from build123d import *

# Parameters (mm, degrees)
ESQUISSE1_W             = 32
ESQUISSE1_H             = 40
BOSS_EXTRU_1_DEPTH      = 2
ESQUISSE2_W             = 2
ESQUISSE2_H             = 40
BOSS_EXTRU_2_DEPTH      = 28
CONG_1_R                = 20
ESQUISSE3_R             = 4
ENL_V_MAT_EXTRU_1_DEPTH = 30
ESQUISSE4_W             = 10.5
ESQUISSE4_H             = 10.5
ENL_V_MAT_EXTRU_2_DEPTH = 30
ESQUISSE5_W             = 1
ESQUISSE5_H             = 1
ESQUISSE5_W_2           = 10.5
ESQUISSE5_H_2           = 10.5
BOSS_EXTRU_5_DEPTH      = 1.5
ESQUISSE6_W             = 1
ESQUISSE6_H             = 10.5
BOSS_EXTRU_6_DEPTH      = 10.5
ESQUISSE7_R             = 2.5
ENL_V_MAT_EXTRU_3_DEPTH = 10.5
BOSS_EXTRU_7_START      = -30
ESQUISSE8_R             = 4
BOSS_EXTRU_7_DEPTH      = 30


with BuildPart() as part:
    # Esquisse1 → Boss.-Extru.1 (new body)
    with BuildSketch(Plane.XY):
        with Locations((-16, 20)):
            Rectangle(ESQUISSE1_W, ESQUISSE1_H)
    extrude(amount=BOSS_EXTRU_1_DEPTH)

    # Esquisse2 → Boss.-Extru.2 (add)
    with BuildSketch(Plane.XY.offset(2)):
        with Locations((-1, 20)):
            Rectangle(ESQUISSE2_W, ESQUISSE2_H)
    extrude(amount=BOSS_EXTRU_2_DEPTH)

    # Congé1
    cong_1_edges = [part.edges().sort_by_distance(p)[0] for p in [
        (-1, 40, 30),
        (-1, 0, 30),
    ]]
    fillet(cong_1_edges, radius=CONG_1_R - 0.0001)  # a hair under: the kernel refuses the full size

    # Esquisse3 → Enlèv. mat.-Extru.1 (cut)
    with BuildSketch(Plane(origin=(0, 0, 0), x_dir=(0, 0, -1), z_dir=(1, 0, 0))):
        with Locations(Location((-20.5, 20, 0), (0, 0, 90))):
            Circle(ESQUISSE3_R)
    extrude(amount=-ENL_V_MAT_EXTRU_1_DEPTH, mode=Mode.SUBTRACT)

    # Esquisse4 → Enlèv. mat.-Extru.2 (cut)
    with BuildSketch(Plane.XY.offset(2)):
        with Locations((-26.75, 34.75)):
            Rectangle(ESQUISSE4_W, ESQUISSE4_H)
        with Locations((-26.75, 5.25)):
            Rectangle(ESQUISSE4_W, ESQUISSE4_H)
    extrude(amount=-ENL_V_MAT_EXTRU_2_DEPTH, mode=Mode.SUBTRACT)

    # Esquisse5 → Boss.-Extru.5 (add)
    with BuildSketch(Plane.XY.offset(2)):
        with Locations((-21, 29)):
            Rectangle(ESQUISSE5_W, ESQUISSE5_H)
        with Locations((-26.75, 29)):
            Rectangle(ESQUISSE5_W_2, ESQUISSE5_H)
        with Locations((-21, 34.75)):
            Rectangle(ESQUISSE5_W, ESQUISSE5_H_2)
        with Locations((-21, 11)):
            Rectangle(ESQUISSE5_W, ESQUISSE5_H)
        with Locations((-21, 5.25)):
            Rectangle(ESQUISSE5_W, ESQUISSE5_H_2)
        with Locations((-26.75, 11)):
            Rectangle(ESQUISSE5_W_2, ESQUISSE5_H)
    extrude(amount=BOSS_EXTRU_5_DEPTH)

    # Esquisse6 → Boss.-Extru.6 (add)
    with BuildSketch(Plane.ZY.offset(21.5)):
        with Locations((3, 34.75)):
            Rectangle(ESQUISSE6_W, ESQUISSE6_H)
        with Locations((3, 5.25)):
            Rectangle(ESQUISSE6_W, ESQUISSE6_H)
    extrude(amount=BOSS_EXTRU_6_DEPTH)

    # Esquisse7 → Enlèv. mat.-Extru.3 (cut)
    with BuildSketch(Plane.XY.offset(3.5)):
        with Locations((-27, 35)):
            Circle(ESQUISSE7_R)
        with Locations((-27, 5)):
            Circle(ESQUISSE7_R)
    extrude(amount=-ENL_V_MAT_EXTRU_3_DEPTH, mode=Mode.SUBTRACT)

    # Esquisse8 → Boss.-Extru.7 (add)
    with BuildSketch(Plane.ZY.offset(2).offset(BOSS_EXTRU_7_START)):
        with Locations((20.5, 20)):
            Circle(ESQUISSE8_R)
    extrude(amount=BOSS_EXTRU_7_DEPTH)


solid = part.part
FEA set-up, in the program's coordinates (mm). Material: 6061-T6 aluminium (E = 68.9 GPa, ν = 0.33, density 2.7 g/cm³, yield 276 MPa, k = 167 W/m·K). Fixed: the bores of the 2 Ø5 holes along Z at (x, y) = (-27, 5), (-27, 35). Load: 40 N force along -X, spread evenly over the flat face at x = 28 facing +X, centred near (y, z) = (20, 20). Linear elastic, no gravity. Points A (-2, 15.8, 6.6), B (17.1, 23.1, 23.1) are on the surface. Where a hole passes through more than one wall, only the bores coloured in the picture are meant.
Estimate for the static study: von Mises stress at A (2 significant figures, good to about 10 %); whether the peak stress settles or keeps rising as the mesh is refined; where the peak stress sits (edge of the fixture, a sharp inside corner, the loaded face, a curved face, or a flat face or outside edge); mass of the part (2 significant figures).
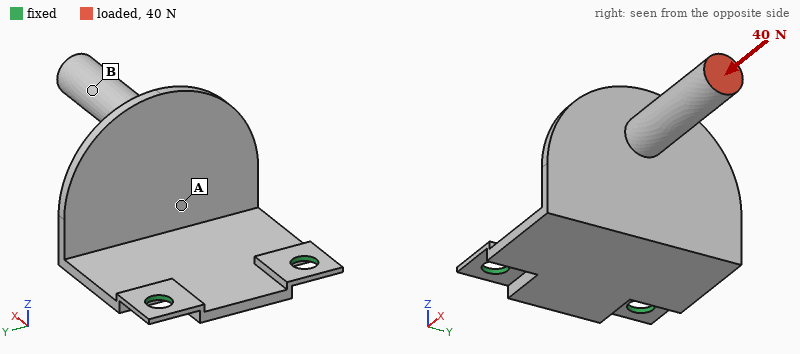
20 MPa
keeps rising
edge of the fixture
15 g
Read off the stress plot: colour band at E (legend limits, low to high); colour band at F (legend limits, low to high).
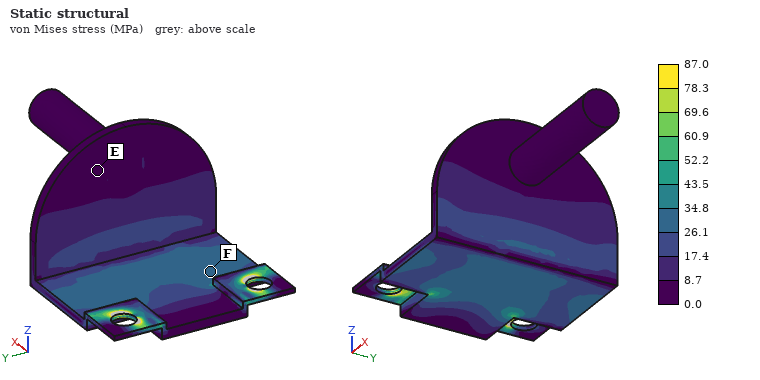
0.0 to 8.7 MPa
26.1 to 34.8 MPa
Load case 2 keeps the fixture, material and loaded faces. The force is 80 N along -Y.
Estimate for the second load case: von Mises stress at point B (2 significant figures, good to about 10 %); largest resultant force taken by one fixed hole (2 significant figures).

14 MPa
150 N
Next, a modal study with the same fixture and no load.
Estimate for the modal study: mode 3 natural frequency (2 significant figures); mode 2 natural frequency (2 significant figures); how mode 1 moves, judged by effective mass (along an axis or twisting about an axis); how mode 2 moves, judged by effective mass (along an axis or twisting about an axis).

1500 Hz
1100 Hz
along Z
along Y
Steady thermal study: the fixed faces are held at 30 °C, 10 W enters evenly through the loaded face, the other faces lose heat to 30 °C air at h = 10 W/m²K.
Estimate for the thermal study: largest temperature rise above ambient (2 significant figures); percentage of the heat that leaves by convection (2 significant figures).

72 K
14 %
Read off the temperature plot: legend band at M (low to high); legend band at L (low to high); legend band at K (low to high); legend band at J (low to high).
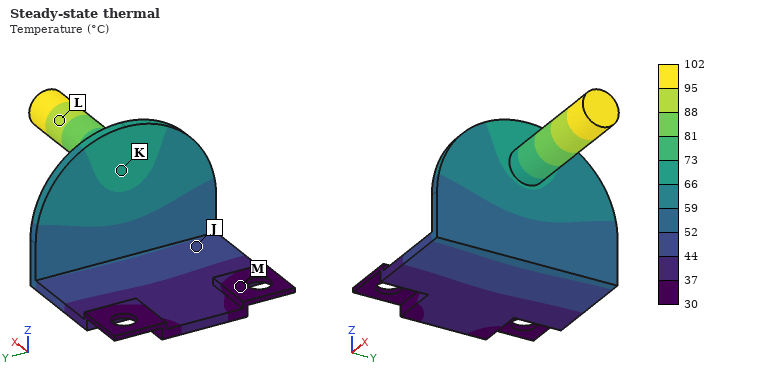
30 to 37 °C
88 to 95 °C
66 to 73 °C
44 to 52 °C
